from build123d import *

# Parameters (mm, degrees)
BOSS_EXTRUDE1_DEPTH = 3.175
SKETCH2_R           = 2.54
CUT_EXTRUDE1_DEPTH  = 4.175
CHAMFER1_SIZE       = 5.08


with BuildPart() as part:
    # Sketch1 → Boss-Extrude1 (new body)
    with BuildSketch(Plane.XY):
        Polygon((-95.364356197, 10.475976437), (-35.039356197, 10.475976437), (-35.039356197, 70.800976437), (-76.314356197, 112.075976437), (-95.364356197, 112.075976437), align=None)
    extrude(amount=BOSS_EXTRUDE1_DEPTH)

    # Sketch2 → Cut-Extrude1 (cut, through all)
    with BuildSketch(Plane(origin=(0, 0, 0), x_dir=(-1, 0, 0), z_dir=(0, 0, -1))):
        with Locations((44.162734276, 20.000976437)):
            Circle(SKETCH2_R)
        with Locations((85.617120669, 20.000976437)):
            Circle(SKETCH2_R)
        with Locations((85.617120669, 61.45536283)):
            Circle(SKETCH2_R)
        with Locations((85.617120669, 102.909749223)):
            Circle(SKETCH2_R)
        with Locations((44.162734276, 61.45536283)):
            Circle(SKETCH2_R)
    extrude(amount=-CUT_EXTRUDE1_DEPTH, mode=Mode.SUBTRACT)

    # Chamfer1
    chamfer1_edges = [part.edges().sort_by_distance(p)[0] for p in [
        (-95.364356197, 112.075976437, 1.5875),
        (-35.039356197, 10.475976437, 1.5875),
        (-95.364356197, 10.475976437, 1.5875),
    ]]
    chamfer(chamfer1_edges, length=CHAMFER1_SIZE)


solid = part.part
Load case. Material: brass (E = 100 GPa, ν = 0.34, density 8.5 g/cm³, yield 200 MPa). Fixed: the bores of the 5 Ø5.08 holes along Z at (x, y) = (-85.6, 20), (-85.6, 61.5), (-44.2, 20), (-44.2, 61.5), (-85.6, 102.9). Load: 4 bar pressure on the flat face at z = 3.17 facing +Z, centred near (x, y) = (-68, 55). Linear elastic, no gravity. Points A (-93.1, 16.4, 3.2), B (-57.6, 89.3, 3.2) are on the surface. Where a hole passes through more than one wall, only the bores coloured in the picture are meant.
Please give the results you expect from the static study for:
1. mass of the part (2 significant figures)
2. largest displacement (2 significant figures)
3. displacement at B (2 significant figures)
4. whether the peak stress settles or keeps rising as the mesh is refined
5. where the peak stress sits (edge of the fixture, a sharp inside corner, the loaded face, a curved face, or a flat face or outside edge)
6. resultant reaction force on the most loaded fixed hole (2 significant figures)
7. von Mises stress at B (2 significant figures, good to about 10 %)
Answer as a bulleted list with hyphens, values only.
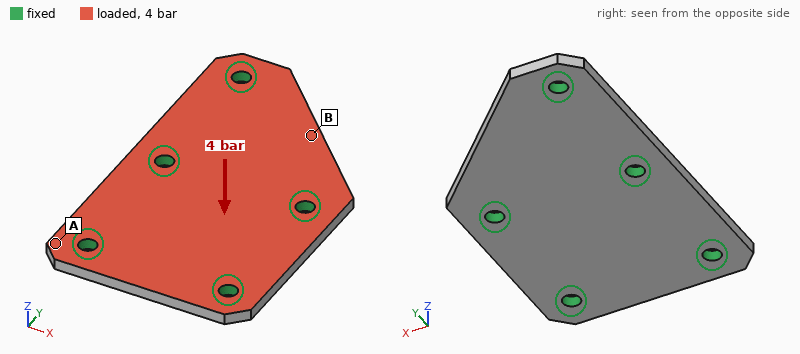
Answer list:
- 140 g
- 49 µm
- 45 µm
- keeps rising
- edge of the fixture
- 510 N
- 27 MPa
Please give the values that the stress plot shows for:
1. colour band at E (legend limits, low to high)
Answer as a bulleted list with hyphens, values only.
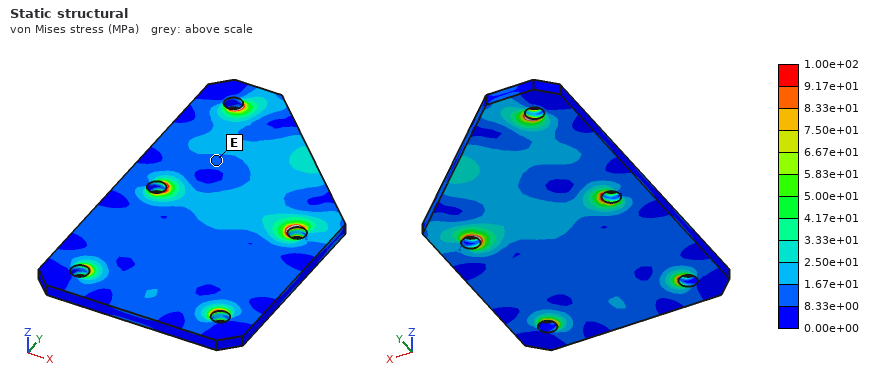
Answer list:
- 8.33e+00 to 1.67e+01 MPa
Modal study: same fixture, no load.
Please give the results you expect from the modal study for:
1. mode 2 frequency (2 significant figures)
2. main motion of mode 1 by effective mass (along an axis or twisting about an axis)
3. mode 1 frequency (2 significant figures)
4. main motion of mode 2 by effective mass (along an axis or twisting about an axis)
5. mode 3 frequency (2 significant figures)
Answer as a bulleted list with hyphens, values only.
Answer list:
- 5100 Hz
- along Z
- 3600 Hz
- along Z
- 6800 Hz
